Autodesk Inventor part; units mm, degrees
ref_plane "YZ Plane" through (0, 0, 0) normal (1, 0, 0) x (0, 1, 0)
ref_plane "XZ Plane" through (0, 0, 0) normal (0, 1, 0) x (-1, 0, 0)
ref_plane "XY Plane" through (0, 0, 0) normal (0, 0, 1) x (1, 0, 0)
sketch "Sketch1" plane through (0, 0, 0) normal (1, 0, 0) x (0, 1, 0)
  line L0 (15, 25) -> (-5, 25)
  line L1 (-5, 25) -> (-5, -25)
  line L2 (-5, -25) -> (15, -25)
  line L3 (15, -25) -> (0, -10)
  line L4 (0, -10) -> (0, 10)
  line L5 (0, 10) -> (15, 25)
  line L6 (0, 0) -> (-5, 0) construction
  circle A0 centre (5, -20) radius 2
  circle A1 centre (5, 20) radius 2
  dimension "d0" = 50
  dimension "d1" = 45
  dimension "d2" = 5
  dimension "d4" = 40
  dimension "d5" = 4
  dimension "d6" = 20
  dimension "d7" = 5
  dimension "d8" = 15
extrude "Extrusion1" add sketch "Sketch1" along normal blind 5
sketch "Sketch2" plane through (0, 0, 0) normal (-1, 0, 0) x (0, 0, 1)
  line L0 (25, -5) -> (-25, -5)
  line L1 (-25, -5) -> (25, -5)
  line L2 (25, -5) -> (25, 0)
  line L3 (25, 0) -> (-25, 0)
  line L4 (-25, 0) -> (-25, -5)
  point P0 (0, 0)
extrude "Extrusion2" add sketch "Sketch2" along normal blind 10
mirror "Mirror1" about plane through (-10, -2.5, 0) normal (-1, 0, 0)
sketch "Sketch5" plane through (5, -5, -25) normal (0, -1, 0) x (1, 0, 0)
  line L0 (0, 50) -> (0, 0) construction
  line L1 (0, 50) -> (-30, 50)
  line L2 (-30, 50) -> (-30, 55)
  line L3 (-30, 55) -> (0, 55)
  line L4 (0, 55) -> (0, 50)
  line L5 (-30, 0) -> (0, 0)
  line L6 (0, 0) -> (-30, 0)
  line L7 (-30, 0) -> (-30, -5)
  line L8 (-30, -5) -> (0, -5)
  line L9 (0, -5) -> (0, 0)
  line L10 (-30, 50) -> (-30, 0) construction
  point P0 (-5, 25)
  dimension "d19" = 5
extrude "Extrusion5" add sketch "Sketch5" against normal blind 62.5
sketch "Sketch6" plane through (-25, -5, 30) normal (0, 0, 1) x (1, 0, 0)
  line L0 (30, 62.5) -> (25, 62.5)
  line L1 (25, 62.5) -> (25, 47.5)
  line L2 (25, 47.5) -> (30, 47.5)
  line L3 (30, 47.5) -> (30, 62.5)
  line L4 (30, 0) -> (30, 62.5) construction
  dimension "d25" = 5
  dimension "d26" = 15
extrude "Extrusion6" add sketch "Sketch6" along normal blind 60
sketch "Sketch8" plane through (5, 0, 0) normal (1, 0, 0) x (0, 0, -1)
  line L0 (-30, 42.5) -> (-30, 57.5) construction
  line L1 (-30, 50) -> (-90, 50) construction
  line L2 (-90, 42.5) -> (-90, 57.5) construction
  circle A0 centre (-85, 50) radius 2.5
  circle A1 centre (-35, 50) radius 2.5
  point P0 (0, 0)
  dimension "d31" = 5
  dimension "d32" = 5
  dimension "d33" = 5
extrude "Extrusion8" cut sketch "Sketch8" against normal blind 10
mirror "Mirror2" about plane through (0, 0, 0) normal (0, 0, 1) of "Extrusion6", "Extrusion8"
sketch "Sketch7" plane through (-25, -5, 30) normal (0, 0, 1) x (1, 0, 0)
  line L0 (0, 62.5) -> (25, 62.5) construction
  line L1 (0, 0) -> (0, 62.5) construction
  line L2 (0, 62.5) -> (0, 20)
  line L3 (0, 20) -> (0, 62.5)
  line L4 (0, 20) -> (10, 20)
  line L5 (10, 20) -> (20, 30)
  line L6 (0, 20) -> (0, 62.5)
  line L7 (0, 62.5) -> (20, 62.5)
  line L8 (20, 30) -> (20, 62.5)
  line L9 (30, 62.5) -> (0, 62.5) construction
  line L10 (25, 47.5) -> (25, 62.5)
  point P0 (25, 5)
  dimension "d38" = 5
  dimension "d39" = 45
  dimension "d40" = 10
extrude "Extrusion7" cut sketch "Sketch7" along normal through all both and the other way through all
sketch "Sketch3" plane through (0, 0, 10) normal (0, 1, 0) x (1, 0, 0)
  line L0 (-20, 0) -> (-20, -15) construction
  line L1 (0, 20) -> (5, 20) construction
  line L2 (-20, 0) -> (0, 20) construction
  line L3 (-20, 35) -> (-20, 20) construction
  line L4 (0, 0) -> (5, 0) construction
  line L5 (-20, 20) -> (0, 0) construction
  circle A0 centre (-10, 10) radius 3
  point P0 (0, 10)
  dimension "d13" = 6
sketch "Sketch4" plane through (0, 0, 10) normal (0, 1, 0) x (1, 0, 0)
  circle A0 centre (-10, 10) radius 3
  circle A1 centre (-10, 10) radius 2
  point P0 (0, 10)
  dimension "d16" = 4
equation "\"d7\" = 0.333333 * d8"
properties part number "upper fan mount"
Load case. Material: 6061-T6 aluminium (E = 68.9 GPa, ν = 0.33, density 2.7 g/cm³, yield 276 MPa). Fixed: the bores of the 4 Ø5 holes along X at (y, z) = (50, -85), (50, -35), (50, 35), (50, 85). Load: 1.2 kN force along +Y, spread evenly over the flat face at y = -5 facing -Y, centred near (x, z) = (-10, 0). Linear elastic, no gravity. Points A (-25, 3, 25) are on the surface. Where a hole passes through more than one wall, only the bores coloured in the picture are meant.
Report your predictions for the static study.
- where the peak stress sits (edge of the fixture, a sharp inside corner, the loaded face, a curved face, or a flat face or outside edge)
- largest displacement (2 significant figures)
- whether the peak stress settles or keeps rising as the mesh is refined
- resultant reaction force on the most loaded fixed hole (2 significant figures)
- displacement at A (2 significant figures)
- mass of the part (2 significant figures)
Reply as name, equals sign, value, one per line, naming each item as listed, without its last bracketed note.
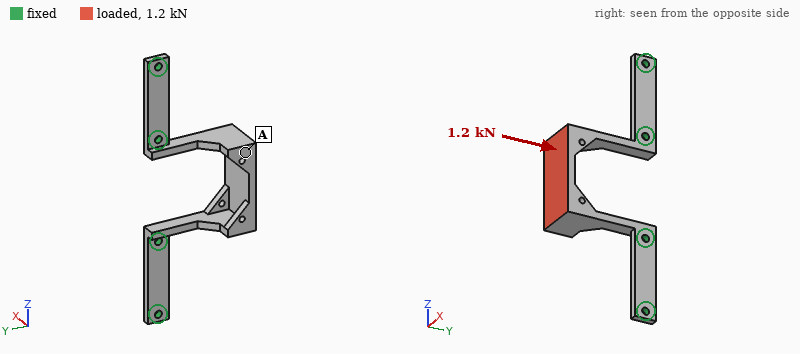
where the peak stress sits = edge of the fixture
largest displacement = 0.47 mm
whether the peak stress settles or keeps rising as the mesh is refined = keeps rising
resultant reaction force on the most loaded fixed hole = 620 N
displacement at A = 0.39 mm
mass of the part = 78 g
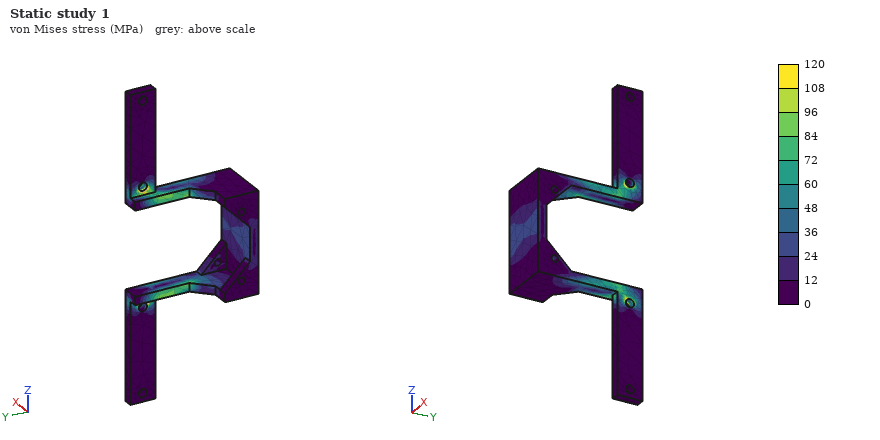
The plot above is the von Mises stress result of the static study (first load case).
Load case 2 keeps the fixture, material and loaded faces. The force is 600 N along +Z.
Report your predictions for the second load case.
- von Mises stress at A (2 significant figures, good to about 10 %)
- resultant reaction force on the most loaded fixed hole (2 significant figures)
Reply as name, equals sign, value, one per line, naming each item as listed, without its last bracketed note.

von Mises stress at A = 12 MPa
resultant reaction force on the most loaded fixed hole = 450 N
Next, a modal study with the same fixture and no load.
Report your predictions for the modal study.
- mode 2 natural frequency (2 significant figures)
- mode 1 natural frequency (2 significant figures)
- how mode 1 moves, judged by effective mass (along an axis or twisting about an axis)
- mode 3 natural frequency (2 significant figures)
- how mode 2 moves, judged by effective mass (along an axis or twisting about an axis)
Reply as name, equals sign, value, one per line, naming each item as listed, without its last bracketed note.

mode 2 natural frequency = 1300 Hz
mode 1 natural frequency = 730 Hz
how mode 1 moves, judged by effective mass = along X
mode 3 natural frequency = 1900 Hz
how mode 2 moves, judged by effective mass = along Z
